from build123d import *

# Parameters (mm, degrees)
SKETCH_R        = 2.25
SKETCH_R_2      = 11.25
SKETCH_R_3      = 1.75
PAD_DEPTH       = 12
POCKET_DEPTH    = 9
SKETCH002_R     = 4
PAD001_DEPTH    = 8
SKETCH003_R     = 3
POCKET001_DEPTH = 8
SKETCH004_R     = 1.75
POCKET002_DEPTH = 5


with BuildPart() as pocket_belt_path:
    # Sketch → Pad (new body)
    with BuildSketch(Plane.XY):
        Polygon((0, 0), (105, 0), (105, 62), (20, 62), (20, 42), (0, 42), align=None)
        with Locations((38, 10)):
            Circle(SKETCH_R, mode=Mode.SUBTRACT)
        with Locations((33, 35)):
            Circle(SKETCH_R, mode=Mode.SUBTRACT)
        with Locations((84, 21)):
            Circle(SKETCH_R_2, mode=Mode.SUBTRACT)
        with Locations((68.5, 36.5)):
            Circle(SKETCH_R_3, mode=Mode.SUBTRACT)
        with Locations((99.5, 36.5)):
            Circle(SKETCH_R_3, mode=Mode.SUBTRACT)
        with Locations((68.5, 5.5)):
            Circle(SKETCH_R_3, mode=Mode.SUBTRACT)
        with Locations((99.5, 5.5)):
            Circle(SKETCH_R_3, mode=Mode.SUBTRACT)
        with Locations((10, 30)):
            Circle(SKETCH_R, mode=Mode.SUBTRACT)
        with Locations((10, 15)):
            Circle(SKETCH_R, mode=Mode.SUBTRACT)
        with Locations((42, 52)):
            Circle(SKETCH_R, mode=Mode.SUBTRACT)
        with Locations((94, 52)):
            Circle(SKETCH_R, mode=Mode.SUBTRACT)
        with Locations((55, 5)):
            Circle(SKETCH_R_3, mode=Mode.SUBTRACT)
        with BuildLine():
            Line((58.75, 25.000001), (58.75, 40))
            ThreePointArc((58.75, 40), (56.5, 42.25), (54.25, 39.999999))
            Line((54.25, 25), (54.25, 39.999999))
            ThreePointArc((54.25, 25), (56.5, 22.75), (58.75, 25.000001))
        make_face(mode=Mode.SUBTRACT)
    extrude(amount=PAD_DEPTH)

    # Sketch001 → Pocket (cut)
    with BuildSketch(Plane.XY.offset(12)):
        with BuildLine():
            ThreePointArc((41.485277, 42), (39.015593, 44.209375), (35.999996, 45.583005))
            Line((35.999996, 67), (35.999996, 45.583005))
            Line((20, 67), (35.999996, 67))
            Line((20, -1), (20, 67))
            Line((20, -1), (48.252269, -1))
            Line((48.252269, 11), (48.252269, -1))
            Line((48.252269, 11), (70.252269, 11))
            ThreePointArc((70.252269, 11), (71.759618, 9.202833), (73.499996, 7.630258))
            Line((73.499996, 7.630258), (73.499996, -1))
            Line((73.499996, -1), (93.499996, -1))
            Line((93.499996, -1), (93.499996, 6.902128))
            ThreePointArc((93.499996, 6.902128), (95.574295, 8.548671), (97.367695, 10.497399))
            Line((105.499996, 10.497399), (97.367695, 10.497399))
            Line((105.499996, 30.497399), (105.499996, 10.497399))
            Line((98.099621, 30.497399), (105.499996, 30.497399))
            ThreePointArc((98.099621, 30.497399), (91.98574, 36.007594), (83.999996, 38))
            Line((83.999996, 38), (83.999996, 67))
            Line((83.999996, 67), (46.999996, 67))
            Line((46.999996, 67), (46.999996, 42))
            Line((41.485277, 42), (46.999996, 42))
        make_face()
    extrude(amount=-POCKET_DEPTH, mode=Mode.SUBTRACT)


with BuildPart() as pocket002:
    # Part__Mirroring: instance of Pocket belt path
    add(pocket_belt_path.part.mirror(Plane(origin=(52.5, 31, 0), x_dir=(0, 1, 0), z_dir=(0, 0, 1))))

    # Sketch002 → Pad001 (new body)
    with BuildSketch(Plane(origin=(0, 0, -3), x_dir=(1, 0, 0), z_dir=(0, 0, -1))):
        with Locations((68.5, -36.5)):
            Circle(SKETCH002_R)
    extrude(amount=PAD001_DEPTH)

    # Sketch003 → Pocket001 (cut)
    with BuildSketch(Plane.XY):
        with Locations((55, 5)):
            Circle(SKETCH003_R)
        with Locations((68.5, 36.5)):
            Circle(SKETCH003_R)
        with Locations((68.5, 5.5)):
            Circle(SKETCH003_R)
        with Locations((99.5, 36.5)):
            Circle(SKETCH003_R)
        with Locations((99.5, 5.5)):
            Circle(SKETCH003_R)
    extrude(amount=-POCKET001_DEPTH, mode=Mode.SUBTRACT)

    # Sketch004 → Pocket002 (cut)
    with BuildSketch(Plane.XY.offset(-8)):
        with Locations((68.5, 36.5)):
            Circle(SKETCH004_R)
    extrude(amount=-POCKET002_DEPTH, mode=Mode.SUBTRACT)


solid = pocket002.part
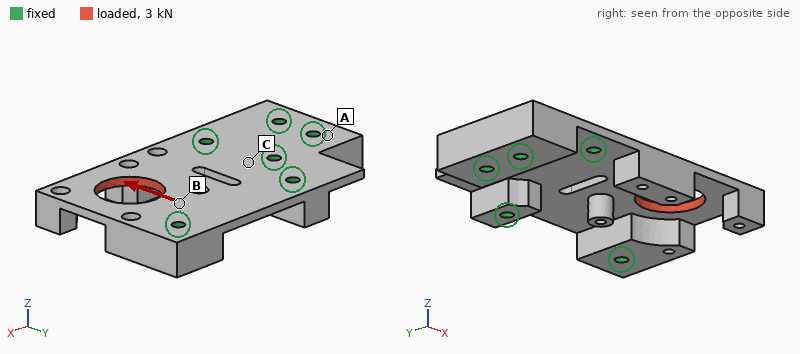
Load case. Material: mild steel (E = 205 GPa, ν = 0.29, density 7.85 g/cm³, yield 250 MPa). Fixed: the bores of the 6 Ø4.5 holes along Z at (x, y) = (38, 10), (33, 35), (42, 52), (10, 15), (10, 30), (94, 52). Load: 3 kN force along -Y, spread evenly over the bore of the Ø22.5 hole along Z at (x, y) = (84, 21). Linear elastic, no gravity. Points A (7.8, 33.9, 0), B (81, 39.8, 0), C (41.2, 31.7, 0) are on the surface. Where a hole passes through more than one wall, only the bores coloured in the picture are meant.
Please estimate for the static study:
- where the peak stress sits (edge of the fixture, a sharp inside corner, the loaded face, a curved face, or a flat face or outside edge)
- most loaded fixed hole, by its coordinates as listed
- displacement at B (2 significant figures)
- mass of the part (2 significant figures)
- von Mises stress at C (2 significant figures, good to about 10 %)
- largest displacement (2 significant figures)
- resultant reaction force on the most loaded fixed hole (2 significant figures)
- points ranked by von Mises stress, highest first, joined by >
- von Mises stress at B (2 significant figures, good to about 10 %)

a curved face
(94, 52)
2.7 µm
260 g
11 MPa
13 µm
2.2 kN
B > C > A
18 MPa
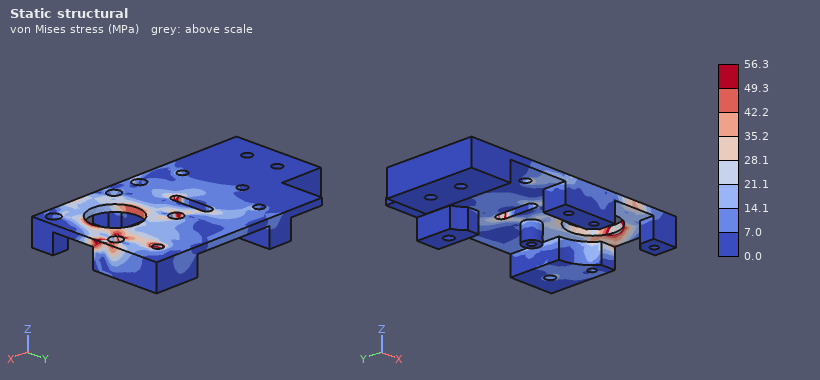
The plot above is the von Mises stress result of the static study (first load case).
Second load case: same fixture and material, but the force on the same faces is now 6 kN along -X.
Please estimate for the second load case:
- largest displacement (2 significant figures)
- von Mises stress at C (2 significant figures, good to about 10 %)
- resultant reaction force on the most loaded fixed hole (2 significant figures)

19 µm
14 MPa
2.3 kN
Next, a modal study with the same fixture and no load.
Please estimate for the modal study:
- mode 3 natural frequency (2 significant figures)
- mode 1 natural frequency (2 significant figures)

6100 Hz
1700 Hz
